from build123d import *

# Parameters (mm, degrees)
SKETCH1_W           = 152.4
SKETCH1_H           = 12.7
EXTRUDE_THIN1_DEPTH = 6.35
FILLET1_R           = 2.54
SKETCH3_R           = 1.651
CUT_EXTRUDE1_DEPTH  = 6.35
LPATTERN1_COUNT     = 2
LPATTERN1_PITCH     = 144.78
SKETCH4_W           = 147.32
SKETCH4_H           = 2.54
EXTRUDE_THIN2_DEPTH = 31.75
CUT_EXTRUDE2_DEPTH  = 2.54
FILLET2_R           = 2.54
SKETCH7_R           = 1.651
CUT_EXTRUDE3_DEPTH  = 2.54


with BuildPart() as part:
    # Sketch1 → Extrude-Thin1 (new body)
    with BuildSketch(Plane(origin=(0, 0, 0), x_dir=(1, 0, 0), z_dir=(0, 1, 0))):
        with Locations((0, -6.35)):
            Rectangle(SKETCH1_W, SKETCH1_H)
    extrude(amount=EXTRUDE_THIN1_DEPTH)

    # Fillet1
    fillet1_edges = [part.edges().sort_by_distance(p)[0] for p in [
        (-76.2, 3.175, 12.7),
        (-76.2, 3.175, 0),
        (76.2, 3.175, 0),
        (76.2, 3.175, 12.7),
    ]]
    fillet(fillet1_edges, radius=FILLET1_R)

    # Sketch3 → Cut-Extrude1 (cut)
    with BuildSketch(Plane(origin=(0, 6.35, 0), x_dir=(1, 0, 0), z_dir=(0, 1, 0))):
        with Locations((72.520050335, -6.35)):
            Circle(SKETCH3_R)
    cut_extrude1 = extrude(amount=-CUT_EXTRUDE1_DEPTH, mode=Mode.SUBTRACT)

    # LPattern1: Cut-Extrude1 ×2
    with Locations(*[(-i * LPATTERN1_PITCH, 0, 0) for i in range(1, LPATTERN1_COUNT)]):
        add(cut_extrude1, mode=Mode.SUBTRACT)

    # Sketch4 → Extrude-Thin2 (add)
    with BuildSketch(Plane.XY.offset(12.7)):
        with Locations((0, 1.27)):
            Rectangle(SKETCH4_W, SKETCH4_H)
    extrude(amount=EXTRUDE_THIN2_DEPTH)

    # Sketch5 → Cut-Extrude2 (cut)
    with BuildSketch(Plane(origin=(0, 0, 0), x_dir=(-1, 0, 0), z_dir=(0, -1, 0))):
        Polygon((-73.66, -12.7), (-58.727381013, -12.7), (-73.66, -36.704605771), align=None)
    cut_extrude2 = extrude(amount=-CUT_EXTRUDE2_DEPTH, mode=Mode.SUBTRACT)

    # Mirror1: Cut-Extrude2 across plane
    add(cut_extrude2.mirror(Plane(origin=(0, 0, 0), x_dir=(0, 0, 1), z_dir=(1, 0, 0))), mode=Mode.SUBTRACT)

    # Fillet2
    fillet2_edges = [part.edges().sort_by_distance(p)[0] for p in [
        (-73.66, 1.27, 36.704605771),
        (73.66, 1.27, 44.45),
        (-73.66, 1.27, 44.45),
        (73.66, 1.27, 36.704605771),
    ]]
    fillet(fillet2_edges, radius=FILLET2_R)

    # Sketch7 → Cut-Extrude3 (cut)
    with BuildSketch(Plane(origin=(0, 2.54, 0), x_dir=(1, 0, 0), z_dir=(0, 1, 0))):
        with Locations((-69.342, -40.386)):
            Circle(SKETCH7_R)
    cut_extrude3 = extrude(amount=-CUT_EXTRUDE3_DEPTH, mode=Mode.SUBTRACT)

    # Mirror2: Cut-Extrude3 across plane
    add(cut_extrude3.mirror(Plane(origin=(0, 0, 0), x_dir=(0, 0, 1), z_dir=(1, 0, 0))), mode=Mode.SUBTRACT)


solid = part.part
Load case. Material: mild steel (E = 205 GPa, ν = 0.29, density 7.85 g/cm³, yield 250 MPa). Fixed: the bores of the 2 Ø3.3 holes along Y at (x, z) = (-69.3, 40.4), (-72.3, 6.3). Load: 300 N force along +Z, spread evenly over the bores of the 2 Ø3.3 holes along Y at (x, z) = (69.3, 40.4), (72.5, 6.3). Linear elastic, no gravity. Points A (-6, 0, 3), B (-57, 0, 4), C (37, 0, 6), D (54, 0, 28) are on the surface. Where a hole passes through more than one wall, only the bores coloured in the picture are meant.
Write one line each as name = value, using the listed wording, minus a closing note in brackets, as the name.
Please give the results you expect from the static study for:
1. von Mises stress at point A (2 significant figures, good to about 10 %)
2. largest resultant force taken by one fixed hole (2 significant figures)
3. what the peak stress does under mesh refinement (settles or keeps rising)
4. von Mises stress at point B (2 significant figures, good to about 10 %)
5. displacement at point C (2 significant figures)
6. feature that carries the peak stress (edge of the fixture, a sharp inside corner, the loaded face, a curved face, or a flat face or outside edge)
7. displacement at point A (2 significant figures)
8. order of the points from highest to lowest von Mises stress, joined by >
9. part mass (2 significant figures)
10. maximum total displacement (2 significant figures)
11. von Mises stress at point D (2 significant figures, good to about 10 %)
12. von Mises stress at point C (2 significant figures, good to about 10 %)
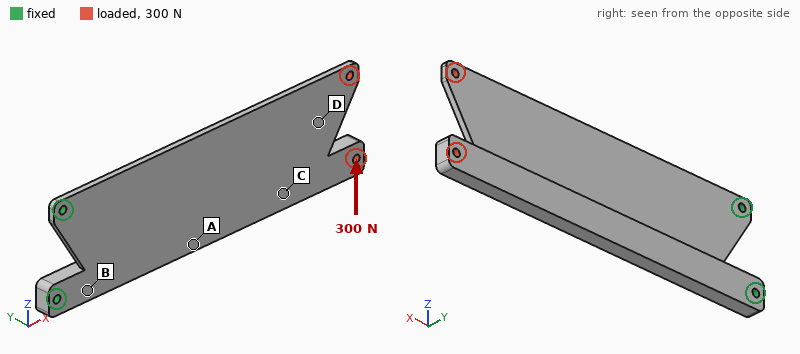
von Mises stress at point A = 25 MPa
largest resultant force taken by one fixed hole = 1.2 kN
what the peak stress does under mesh refinement = keeps rising
von Mises stress at point B = 40 MPa
displacement at point C = 0.18 mm
feature that carries the peak stress = edge of the fixture
displacement at point A = 0.075 mm
order of the points from highest to lowest von Mises stress, joined by > = B > A > C > D
part mass = 180 g
maximum total displacement = 0.29 mm
von Mises stress at point D = 5.4 MPa
von Mises stress at point C = 11 MPa
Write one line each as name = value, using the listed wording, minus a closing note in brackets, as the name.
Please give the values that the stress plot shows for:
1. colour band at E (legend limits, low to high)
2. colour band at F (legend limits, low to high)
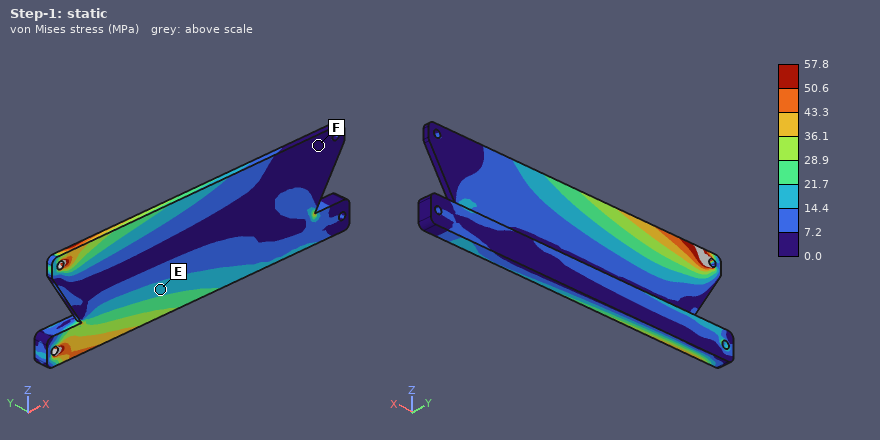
colour band at E = 14.4 to 21.7 MPa
colour band at F = 0.0 to 7.2 MPa
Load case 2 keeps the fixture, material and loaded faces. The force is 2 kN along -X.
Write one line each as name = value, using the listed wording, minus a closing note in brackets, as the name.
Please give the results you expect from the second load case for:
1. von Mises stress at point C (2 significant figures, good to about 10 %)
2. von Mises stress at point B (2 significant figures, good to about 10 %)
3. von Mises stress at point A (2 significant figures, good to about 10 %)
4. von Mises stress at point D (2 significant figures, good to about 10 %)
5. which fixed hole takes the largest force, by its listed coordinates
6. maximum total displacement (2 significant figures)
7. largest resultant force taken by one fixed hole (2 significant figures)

von Mises stress at point C = 9.7 MPa
von Mises stress at point B = 14 MPa
von Mises stress at point A = 8.2 MPa
von Mises stress at point D = 6.4 MPa
which fixed hole takes the largest force, by its listed coordinates = (-72.3, 6.3)
maximum total displacement = 73 µm
largest resultant force taken by one fixed hole = 1.4 kN
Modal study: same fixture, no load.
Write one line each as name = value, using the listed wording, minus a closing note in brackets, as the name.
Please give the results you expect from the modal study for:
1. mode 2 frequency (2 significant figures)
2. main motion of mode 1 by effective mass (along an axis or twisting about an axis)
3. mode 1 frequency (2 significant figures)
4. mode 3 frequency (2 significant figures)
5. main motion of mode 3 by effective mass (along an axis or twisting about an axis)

mode 2 frequency = 960 Hz
main motion of mode 1 by effective mass = along Y
mode 1 frequency = 190 Hz
mode 3 frequency = 1200 Hz
main motion of mode 3 by effective mass = along Y
